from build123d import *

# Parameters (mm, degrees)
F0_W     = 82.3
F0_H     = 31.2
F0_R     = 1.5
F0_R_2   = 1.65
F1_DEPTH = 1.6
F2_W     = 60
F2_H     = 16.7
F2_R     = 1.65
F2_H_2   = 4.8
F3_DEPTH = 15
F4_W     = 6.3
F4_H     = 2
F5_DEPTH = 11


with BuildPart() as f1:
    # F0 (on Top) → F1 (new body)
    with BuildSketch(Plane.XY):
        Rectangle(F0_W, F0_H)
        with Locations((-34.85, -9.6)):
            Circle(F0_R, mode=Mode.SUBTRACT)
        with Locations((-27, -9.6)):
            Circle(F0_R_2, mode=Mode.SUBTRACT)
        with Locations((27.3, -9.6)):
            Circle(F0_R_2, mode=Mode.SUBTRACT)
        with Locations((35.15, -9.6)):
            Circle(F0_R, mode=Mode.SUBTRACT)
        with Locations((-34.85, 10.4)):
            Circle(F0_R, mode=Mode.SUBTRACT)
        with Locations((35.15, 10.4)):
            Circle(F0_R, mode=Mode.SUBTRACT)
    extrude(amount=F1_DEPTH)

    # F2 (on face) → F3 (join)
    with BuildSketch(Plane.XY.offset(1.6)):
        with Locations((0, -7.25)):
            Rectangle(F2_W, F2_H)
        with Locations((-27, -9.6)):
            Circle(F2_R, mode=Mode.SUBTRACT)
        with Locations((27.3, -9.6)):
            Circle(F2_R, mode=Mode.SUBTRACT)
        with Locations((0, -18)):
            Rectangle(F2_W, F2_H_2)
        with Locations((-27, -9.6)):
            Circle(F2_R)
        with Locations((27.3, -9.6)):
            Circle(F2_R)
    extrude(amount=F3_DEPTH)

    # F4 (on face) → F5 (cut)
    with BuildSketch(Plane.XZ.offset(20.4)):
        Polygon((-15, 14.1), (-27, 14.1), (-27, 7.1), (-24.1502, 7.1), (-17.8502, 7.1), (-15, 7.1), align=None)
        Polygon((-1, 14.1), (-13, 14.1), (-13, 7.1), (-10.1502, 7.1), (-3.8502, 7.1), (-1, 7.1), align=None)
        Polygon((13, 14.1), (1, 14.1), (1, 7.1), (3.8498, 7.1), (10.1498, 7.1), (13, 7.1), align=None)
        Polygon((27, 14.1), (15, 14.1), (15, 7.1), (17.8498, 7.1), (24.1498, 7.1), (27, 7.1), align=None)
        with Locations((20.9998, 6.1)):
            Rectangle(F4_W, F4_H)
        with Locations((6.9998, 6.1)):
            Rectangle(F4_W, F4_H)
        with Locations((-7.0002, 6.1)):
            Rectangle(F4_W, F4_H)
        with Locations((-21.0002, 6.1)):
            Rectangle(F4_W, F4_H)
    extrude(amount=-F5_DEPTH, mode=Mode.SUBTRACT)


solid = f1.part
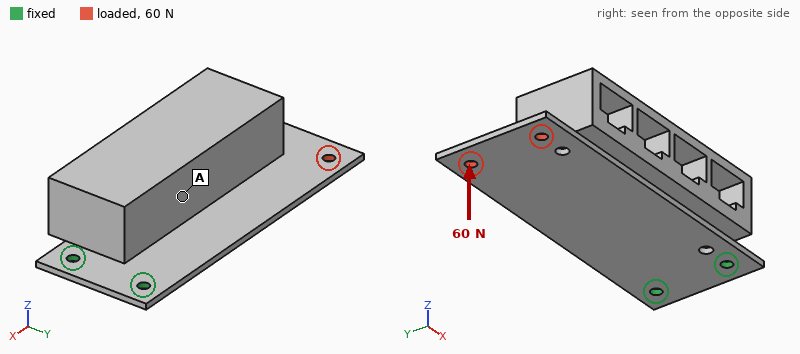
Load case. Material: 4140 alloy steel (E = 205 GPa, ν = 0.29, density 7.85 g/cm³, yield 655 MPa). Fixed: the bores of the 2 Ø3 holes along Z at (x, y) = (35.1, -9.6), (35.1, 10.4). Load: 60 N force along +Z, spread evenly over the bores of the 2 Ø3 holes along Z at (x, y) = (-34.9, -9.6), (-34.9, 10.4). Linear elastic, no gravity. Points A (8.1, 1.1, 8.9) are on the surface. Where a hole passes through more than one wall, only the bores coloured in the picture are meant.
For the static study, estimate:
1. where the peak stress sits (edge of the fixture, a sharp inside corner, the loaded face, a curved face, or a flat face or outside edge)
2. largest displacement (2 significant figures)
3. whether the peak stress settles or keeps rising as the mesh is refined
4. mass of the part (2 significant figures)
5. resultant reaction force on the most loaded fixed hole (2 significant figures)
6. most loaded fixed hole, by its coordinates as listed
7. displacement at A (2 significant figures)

edge of the fixture
0.92 mm
keeps rising
150 g
44 N
(35.1, 10.4)
0.31 mm
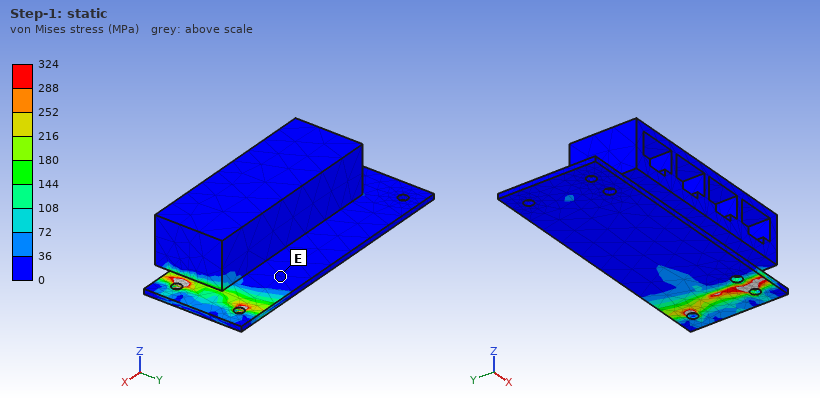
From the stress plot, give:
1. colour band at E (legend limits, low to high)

0 to 36 MPa
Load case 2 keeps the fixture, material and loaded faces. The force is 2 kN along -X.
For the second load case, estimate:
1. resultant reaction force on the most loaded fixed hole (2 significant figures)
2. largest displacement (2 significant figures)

1.0 kN
39 µm
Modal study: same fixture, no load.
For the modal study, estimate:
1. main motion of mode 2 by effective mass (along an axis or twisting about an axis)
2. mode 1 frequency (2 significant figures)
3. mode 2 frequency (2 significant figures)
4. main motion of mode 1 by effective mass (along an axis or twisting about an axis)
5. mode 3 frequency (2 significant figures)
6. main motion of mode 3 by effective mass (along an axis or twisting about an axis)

along Y
190 Hz
1500 Hz
along Z
2600 Hz
along Y
